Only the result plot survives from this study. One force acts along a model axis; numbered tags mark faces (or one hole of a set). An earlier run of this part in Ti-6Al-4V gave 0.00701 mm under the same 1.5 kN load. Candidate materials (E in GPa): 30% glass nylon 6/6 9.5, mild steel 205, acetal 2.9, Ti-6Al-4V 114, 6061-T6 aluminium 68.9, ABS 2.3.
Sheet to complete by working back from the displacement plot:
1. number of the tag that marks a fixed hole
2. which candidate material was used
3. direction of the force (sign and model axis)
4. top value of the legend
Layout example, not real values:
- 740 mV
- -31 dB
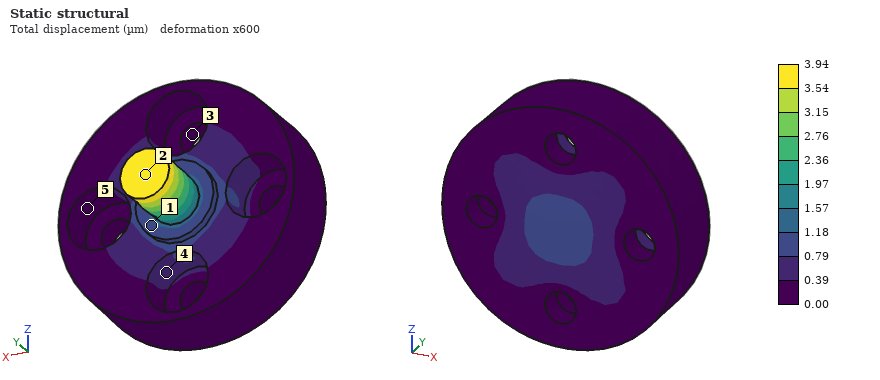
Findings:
- 3
- mild steel
- -Y
- 3.94 µm
